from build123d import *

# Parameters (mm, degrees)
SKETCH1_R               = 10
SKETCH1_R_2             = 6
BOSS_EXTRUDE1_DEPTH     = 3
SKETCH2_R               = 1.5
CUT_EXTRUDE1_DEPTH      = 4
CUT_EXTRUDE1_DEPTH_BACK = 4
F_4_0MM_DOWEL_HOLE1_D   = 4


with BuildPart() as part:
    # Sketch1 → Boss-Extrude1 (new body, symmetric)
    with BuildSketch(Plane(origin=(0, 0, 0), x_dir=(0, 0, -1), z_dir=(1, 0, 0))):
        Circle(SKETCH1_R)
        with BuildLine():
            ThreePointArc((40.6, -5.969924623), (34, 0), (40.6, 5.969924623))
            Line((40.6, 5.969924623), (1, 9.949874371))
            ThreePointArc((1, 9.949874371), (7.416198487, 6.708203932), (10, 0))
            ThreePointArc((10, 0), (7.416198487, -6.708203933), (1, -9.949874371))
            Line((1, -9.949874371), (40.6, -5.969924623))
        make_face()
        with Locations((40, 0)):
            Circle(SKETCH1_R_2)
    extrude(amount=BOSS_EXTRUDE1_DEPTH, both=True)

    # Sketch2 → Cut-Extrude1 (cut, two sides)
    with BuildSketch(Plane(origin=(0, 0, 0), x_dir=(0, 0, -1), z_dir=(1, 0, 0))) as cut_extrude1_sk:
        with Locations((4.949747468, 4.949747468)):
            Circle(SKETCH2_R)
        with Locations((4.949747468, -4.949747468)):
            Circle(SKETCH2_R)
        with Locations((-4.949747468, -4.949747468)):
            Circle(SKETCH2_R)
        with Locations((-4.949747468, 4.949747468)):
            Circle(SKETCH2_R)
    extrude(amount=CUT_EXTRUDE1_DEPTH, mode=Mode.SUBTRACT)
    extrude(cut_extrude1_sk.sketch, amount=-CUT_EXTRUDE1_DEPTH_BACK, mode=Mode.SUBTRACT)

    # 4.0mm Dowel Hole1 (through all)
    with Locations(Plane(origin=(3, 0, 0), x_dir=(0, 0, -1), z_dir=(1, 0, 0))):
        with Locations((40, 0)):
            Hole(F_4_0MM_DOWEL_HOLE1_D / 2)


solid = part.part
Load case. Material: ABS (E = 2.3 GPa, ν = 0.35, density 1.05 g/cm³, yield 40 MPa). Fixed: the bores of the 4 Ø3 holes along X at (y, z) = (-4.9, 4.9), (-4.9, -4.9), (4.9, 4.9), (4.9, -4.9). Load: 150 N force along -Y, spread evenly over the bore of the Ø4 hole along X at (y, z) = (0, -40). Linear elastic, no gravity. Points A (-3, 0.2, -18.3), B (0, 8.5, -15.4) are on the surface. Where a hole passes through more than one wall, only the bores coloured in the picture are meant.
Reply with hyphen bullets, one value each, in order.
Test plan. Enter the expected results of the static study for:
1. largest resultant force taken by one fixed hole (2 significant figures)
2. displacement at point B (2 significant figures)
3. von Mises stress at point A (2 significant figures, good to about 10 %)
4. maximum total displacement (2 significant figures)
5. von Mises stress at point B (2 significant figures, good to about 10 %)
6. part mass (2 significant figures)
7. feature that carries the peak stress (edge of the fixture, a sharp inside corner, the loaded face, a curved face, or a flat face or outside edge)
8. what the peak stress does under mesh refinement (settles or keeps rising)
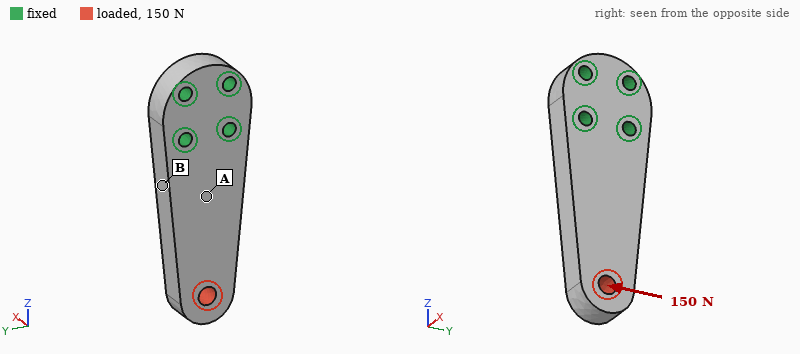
- 390 N
- 0.088 mm
- 3.0 MPa
- 0.57 mm
- 13 MPa
- 5.1 g
- edge of the fixture
- keeps rising
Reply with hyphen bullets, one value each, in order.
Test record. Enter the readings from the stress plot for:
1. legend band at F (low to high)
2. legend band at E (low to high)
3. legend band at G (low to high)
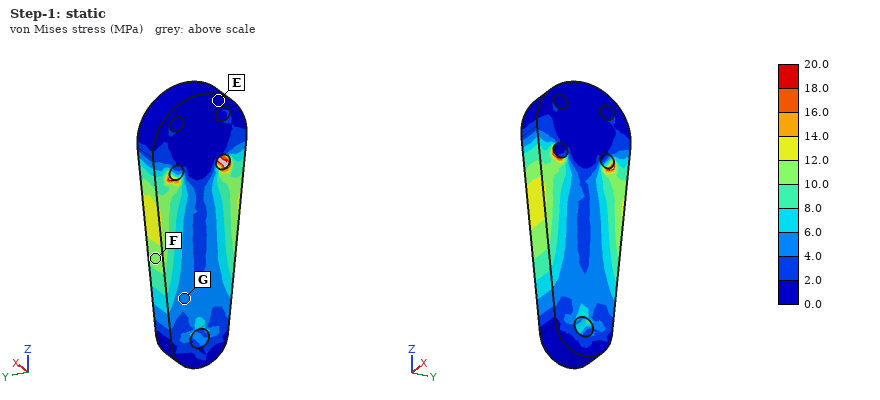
- 10.0 to 12.0 MPa
- 0.0 to 2.0 MPa
- 4.0 to 6.0 MPa
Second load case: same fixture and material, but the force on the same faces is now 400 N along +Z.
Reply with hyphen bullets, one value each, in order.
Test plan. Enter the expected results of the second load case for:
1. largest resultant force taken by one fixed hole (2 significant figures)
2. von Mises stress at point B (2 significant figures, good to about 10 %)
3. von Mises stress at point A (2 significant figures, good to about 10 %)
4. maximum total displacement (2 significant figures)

- 180 N
- 3.7 MPa
- 4.2 MPa
- 84 µm
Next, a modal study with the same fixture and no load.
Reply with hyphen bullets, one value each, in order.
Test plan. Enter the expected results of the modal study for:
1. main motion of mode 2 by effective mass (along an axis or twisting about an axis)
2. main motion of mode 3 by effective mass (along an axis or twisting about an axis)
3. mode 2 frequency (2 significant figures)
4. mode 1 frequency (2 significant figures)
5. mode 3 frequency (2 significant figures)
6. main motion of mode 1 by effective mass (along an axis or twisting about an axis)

- along Y
- twisting about Z
- 2700 Hz
- 1100 Hz
- 5000 Hz
- along X
